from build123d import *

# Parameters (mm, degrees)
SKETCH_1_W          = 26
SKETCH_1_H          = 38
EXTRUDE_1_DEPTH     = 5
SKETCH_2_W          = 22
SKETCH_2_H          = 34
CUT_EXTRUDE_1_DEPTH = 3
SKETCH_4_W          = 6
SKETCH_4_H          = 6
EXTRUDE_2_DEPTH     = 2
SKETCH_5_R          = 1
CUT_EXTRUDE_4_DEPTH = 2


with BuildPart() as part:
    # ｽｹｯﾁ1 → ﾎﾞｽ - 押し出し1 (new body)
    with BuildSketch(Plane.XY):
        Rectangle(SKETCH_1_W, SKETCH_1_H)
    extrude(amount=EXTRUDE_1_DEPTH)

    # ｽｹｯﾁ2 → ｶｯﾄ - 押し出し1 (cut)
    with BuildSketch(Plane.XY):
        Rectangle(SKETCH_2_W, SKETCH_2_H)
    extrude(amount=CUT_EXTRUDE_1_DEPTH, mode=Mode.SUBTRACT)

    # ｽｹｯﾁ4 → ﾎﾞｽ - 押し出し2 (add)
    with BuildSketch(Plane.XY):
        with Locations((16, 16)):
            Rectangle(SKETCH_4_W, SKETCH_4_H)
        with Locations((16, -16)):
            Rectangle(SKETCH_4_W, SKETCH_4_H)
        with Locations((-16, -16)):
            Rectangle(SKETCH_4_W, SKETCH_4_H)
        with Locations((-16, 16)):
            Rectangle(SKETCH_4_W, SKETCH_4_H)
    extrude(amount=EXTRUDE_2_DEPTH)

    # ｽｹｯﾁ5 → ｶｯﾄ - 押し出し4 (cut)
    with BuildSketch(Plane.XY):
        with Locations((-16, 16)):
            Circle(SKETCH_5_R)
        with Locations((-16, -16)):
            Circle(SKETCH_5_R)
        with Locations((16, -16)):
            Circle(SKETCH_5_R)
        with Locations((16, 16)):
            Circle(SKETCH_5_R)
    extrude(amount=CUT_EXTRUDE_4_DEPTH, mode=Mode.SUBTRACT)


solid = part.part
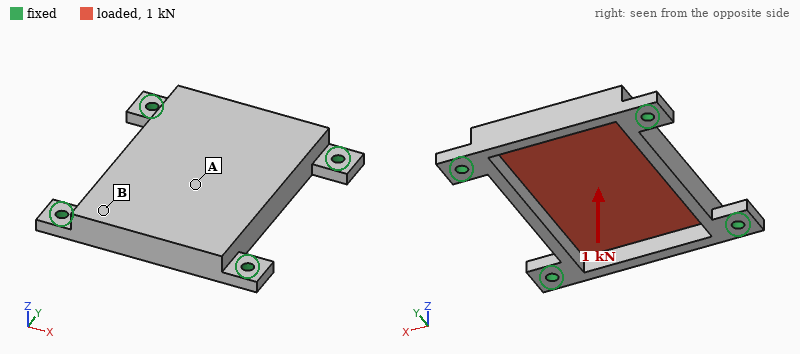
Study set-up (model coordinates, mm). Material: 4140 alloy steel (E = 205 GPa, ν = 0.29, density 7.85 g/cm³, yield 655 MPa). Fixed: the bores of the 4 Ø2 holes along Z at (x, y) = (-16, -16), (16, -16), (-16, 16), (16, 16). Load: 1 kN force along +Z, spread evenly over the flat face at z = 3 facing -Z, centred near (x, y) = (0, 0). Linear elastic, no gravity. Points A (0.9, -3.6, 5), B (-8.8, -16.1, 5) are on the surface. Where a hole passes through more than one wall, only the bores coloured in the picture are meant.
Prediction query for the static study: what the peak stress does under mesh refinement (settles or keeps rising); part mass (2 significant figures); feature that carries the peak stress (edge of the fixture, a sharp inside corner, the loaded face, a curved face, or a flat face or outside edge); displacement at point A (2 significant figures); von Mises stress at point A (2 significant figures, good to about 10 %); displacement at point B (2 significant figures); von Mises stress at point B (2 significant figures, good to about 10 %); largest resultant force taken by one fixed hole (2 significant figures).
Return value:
keeps rising
23 g
edge of the fixture
25 µm
69 MPa
5.2 µm
29 MPa
480 N
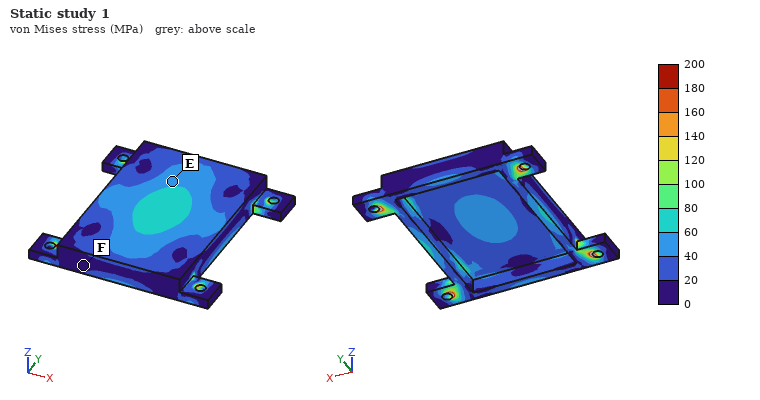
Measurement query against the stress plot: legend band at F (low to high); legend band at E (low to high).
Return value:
0 to 20 MPa
40 to 60 MPa
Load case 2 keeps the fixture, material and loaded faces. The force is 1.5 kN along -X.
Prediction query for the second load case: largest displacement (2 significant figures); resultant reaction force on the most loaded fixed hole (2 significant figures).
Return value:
7.0 µm
380 N
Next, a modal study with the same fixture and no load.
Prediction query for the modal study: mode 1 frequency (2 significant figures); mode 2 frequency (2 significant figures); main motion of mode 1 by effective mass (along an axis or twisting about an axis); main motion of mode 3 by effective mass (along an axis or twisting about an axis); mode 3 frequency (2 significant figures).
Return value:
10 kHz
15 kHz
along Z
twisting about X
17 kHz
